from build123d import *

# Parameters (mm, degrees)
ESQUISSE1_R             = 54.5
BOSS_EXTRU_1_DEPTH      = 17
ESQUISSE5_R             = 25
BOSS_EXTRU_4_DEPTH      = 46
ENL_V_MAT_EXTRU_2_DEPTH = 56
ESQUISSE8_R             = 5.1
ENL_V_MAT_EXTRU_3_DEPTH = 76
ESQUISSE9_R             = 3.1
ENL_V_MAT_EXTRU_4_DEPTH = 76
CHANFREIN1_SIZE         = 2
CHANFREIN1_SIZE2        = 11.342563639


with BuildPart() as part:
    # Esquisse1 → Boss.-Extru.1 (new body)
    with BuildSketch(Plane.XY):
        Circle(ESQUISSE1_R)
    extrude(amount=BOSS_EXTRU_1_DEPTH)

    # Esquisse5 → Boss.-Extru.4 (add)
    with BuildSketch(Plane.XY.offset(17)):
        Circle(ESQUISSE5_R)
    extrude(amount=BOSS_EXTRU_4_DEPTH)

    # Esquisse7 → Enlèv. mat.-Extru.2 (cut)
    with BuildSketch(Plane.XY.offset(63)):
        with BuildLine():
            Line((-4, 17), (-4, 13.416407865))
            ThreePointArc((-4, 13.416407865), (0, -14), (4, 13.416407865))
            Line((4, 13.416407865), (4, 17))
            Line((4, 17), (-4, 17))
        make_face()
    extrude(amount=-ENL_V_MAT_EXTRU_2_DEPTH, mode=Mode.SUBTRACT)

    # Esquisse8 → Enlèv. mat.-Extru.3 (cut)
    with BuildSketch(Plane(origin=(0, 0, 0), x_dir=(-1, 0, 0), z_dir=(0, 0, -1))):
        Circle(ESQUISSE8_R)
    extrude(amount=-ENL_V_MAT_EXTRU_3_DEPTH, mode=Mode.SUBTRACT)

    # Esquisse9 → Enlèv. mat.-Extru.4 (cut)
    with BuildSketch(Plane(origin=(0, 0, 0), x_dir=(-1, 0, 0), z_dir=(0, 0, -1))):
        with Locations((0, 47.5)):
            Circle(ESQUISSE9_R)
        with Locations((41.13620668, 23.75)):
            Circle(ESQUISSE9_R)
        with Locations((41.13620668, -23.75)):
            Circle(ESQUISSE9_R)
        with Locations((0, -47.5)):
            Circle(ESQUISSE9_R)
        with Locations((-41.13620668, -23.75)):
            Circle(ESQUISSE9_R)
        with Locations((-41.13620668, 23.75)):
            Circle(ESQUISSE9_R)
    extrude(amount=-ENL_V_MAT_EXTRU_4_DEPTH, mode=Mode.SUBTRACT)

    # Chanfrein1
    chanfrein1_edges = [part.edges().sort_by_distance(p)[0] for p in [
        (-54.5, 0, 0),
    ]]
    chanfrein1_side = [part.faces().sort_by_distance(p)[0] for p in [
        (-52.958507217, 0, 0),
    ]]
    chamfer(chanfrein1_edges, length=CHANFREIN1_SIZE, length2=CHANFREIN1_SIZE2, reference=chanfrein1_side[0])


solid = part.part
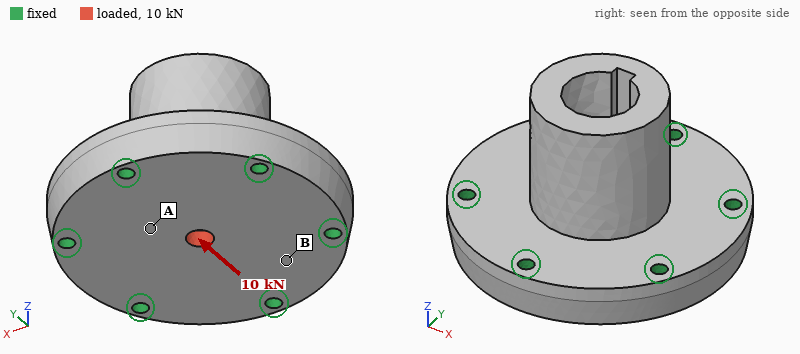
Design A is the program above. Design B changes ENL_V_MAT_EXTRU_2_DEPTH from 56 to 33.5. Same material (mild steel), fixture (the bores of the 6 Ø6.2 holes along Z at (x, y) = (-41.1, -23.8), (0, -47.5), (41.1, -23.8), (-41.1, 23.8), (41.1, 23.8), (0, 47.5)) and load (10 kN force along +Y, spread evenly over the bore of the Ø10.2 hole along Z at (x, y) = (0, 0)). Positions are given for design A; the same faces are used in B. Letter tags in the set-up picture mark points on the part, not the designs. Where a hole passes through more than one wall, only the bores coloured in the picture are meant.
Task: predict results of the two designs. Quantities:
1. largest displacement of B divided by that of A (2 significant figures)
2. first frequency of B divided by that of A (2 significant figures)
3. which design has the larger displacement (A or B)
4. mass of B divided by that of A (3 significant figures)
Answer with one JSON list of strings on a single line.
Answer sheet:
["0.59", "1.0", "A", "1.06"]
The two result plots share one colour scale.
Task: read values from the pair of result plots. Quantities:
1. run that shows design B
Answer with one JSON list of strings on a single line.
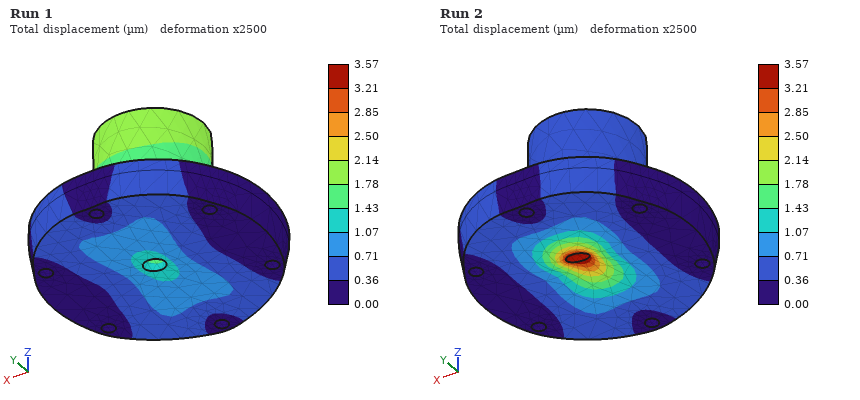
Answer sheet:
["Run 1"]
